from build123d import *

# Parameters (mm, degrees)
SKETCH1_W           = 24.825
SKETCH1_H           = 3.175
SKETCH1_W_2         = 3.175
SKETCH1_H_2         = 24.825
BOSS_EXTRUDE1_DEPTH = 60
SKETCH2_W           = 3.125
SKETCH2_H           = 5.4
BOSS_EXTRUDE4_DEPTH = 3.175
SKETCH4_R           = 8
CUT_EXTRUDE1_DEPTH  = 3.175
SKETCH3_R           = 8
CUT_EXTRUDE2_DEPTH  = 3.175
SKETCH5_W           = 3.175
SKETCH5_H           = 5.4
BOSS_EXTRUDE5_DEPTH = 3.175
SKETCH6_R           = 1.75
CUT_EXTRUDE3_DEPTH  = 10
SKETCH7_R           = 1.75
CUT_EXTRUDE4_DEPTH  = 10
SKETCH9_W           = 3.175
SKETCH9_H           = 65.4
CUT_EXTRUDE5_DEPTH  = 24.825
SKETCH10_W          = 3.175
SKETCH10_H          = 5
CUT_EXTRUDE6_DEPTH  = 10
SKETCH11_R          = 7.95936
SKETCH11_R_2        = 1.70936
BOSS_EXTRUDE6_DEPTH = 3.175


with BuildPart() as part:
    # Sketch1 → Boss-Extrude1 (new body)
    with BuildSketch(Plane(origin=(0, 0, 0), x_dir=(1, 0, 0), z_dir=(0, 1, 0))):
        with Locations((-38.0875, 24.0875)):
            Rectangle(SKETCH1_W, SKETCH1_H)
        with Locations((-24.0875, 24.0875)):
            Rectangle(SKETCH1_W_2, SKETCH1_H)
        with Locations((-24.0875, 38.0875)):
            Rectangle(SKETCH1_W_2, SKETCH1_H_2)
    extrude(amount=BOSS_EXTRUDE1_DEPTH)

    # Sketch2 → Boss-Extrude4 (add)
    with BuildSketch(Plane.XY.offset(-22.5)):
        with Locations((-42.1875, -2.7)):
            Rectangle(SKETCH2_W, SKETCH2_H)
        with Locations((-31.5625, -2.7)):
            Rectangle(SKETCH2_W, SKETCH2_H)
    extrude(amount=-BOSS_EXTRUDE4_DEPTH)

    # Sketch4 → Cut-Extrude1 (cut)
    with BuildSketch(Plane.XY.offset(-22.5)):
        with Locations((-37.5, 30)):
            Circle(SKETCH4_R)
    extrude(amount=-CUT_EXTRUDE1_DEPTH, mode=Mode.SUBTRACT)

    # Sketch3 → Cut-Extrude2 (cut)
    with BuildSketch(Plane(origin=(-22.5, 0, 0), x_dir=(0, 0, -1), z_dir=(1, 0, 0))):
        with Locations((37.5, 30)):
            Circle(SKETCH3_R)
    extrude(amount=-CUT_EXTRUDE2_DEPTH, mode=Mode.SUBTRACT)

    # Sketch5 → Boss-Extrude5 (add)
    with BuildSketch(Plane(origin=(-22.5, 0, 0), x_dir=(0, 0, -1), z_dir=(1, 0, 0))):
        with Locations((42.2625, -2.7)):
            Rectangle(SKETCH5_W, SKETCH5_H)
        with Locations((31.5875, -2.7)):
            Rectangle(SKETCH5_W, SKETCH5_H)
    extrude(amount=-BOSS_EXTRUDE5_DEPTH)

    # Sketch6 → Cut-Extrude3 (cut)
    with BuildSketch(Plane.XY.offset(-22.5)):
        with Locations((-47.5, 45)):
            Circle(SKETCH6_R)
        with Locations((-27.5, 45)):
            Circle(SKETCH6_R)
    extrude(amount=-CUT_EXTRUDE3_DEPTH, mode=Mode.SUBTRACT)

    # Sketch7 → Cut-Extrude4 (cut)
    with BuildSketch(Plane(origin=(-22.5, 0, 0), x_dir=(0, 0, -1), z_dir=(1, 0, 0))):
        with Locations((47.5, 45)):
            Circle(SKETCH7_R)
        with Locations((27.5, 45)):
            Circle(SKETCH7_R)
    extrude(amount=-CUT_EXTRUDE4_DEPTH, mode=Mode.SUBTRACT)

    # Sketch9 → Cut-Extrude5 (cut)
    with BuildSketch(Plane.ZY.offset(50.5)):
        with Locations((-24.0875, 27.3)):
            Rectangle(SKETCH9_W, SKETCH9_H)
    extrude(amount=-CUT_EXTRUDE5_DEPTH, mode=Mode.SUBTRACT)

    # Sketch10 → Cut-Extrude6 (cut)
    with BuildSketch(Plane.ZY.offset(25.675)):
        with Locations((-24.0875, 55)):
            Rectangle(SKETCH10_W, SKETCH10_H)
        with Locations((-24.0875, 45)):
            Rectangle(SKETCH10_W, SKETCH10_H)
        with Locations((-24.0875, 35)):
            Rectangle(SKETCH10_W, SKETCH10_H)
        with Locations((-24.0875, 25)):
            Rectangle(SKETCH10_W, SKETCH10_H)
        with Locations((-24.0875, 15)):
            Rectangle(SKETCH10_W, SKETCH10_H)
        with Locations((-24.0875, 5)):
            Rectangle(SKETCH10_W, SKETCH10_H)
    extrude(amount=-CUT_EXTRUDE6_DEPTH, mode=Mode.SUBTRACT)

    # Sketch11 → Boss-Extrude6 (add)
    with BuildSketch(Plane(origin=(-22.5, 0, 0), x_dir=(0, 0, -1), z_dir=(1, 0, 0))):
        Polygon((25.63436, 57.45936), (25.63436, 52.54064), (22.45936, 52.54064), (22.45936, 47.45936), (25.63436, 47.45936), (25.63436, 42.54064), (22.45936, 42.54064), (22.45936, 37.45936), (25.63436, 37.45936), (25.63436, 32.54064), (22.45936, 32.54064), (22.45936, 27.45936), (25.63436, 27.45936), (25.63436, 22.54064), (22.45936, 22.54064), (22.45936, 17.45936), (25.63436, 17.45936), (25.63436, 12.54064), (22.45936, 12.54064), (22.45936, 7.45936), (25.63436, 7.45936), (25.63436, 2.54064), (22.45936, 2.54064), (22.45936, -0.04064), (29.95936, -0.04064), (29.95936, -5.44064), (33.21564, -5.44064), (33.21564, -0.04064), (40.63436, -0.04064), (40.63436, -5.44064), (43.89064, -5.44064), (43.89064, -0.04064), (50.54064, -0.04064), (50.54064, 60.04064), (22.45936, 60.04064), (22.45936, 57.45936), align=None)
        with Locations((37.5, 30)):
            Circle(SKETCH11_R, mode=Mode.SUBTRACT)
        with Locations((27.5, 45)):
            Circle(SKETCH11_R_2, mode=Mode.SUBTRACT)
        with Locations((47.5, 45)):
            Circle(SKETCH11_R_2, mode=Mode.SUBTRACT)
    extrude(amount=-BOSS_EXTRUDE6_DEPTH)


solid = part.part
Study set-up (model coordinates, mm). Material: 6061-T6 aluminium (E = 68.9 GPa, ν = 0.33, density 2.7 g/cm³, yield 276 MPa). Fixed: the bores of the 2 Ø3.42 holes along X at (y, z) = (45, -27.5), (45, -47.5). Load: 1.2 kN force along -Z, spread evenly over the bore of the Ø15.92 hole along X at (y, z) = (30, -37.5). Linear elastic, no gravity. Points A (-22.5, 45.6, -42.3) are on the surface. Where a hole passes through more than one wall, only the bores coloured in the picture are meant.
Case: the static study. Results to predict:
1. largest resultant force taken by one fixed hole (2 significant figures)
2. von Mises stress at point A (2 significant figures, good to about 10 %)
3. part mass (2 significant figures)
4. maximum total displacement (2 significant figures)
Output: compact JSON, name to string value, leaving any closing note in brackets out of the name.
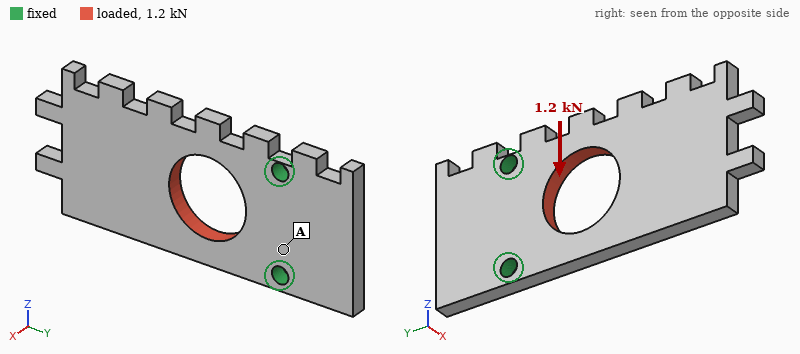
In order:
{"largest resultant force taken by one fixed hole": "1.0 kN", "von Mises stress at point A": "22 MPa", "part mass": "12 g", "maximum total displacement": "77 µm"}
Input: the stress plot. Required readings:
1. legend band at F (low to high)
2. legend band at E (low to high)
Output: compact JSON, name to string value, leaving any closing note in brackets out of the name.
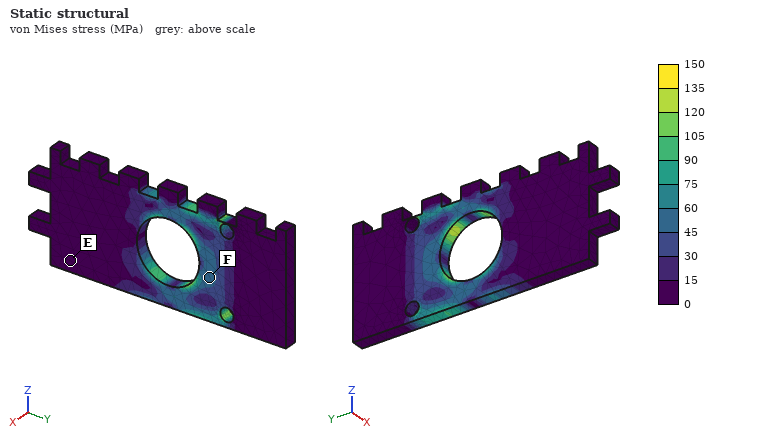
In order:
{"legend band at F": "45 to 60 MPa", "legend band at E": "0 to 15 MPa"}
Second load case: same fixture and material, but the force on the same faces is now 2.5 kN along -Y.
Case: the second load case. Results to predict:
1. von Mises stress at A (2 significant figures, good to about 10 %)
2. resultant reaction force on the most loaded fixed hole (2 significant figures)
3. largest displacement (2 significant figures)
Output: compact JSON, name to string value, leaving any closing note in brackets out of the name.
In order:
{"von Mises stress at A": "11 MPa", "resultant reaction force on the most loaded fixed hole": "1.3 kN", "largest displacement": "18 µm"}
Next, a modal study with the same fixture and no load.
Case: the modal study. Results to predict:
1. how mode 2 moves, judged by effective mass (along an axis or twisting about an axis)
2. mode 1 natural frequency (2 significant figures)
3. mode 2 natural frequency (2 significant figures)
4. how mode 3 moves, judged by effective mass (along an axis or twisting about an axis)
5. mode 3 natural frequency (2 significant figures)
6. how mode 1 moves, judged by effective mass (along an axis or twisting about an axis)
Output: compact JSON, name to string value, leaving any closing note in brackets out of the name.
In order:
{"how mode 2 moves, judged by effective mass": "twisting about Y", "mode 1 natural frequency": "910 Hz", "mode 2 natural frequency": "3700 Hz", "how mode 3 moves, judged by effective mass": "along Z", "mode 3 natural frequency": "5500 Hz", "how mode 1 moves, judged by effective mass": "along X"}
